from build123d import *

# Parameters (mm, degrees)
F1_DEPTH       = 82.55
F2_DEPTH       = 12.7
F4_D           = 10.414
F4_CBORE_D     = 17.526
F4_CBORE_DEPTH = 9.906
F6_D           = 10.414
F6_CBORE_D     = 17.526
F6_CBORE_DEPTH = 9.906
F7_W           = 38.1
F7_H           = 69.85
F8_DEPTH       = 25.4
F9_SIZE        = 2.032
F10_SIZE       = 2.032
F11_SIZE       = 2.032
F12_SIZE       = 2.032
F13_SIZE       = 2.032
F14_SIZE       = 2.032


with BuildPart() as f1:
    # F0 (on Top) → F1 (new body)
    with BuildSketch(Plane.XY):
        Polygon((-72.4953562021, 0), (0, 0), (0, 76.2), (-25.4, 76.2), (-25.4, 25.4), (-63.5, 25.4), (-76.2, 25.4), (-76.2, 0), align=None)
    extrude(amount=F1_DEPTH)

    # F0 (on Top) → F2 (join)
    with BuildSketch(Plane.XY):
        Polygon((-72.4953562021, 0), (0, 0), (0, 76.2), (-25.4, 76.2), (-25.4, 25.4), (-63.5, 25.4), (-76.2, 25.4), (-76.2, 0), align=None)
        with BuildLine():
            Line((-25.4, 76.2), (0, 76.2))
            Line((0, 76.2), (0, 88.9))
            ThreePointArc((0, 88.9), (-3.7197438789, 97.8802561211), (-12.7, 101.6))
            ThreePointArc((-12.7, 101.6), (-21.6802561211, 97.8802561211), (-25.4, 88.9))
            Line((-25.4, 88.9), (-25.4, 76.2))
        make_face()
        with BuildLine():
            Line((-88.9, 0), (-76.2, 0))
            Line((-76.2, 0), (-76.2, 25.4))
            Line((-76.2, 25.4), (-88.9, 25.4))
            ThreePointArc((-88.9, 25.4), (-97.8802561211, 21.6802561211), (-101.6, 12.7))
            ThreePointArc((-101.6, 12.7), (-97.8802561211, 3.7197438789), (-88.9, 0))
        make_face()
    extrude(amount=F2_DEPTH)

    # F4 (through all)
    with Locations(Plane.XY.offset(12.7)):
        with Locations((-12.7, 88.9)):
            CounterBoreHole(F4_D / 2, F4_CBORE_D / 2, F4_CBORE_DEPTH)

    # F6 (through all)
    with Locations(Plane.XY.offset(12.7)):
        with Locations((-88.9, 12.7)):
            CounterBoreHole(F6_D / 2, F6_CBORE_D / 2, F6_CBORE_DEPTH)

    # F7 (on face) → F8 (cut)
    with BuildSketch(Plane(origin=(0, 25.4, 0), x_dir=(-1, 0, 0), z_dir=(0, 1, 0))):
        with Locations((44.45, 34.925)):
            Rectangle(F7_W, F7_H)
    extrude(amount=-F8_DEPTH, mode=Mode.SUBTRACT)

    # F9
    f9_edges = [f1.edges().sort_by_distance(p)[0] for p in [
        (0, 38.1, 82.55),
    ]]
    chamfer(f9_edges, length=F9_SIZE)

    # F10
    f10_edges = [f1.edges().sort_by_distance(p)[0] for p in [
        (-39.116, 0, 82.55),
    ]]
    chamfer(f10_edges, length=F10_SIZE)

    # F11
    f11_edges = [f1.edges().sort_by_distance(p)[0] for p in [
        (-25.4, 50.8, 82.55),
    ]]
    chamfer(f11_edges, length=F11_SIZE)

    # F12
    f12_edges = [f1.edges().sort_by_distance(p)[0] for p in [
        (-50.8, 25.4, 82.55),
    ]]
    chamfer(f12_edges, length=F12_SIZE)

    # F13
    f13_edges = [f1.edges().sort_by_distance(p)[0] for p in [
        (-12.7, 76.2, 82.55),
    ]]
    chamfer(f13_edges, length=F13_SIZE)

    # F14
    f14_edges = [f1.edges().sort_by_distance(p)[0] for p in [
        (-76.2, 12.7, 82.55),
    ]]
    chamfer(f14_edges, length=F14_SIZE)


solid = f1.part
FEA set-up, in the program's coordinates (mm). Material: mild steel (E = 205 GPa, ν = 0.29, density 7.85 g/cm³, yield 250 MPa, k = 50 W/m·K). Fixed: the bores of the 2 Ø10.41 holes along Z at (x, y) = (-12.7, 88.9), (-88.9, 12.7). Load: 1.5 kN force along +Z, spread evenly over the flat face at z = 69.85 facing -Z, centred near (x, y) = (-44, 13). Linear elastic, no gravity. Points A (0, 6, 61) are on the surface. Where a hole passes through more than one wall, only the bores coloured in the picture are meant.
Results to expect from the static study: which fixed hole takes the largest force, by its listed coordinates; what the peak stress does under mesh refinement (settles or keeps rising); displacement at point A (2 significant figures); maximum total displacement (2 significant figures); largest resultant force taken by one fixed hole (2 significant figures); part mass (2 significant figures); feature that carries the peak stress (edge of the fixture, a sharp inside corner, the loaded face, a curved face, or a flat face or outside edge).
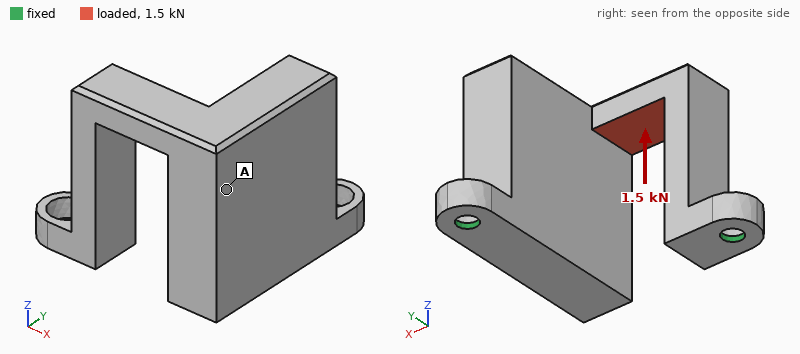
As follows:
(-88.9, 12.7)
keeps rising
0.13 mm
0.16 mm
1.1 kN
1.6 kg
edge of the fixture
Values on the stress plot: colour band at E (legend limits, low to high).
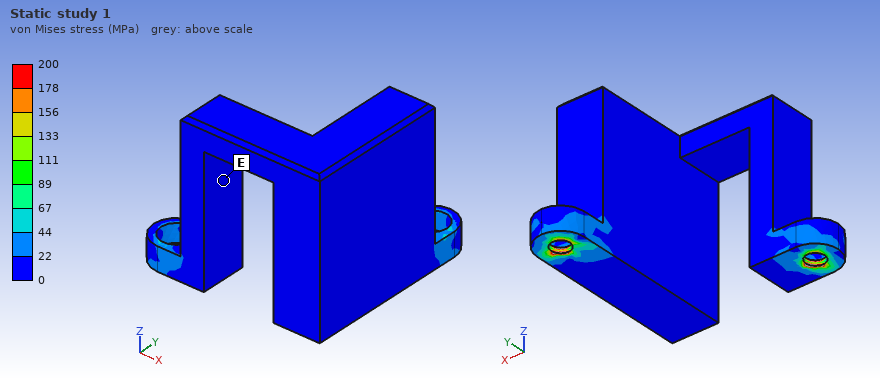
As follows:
0 to 22 MPa
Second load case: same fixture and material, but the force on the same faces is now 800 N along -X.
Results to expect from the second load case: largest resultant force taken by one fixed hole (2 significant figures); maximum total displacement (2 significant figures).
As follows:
600 N
0.13 mm
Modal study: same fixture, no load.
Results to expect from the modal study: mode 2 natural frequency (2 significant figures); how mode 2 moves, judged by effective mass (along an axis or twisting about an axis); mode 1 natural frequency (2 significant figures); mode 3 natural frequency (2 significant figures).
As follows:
1000 Hz
along X
370 Hz
1600 Hz
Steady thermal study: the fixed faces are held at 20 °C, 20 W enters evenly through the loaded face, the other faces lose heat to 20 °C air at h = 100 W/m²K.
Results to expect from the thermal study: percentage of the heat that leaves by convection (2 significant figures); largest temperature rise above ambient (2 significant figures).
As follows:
88 %
21 K
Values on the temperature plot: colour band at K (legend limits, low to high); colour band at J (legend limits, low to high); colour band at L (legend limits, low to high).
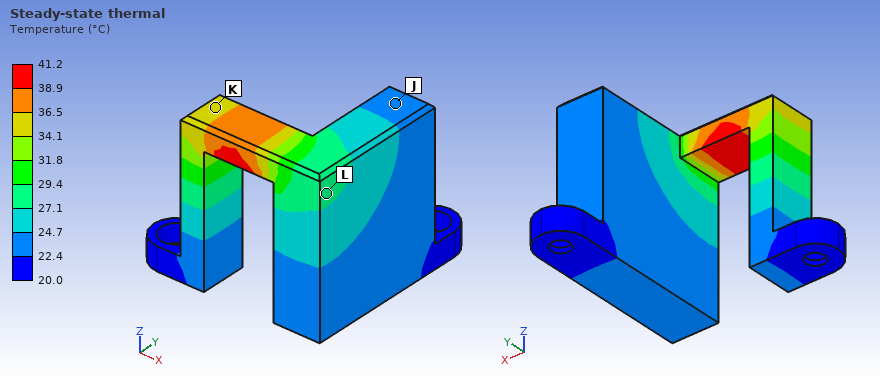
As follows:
34.1 to 36.5 °C
22.4 to 24.7 °C
27.1 to 29.4 °C
